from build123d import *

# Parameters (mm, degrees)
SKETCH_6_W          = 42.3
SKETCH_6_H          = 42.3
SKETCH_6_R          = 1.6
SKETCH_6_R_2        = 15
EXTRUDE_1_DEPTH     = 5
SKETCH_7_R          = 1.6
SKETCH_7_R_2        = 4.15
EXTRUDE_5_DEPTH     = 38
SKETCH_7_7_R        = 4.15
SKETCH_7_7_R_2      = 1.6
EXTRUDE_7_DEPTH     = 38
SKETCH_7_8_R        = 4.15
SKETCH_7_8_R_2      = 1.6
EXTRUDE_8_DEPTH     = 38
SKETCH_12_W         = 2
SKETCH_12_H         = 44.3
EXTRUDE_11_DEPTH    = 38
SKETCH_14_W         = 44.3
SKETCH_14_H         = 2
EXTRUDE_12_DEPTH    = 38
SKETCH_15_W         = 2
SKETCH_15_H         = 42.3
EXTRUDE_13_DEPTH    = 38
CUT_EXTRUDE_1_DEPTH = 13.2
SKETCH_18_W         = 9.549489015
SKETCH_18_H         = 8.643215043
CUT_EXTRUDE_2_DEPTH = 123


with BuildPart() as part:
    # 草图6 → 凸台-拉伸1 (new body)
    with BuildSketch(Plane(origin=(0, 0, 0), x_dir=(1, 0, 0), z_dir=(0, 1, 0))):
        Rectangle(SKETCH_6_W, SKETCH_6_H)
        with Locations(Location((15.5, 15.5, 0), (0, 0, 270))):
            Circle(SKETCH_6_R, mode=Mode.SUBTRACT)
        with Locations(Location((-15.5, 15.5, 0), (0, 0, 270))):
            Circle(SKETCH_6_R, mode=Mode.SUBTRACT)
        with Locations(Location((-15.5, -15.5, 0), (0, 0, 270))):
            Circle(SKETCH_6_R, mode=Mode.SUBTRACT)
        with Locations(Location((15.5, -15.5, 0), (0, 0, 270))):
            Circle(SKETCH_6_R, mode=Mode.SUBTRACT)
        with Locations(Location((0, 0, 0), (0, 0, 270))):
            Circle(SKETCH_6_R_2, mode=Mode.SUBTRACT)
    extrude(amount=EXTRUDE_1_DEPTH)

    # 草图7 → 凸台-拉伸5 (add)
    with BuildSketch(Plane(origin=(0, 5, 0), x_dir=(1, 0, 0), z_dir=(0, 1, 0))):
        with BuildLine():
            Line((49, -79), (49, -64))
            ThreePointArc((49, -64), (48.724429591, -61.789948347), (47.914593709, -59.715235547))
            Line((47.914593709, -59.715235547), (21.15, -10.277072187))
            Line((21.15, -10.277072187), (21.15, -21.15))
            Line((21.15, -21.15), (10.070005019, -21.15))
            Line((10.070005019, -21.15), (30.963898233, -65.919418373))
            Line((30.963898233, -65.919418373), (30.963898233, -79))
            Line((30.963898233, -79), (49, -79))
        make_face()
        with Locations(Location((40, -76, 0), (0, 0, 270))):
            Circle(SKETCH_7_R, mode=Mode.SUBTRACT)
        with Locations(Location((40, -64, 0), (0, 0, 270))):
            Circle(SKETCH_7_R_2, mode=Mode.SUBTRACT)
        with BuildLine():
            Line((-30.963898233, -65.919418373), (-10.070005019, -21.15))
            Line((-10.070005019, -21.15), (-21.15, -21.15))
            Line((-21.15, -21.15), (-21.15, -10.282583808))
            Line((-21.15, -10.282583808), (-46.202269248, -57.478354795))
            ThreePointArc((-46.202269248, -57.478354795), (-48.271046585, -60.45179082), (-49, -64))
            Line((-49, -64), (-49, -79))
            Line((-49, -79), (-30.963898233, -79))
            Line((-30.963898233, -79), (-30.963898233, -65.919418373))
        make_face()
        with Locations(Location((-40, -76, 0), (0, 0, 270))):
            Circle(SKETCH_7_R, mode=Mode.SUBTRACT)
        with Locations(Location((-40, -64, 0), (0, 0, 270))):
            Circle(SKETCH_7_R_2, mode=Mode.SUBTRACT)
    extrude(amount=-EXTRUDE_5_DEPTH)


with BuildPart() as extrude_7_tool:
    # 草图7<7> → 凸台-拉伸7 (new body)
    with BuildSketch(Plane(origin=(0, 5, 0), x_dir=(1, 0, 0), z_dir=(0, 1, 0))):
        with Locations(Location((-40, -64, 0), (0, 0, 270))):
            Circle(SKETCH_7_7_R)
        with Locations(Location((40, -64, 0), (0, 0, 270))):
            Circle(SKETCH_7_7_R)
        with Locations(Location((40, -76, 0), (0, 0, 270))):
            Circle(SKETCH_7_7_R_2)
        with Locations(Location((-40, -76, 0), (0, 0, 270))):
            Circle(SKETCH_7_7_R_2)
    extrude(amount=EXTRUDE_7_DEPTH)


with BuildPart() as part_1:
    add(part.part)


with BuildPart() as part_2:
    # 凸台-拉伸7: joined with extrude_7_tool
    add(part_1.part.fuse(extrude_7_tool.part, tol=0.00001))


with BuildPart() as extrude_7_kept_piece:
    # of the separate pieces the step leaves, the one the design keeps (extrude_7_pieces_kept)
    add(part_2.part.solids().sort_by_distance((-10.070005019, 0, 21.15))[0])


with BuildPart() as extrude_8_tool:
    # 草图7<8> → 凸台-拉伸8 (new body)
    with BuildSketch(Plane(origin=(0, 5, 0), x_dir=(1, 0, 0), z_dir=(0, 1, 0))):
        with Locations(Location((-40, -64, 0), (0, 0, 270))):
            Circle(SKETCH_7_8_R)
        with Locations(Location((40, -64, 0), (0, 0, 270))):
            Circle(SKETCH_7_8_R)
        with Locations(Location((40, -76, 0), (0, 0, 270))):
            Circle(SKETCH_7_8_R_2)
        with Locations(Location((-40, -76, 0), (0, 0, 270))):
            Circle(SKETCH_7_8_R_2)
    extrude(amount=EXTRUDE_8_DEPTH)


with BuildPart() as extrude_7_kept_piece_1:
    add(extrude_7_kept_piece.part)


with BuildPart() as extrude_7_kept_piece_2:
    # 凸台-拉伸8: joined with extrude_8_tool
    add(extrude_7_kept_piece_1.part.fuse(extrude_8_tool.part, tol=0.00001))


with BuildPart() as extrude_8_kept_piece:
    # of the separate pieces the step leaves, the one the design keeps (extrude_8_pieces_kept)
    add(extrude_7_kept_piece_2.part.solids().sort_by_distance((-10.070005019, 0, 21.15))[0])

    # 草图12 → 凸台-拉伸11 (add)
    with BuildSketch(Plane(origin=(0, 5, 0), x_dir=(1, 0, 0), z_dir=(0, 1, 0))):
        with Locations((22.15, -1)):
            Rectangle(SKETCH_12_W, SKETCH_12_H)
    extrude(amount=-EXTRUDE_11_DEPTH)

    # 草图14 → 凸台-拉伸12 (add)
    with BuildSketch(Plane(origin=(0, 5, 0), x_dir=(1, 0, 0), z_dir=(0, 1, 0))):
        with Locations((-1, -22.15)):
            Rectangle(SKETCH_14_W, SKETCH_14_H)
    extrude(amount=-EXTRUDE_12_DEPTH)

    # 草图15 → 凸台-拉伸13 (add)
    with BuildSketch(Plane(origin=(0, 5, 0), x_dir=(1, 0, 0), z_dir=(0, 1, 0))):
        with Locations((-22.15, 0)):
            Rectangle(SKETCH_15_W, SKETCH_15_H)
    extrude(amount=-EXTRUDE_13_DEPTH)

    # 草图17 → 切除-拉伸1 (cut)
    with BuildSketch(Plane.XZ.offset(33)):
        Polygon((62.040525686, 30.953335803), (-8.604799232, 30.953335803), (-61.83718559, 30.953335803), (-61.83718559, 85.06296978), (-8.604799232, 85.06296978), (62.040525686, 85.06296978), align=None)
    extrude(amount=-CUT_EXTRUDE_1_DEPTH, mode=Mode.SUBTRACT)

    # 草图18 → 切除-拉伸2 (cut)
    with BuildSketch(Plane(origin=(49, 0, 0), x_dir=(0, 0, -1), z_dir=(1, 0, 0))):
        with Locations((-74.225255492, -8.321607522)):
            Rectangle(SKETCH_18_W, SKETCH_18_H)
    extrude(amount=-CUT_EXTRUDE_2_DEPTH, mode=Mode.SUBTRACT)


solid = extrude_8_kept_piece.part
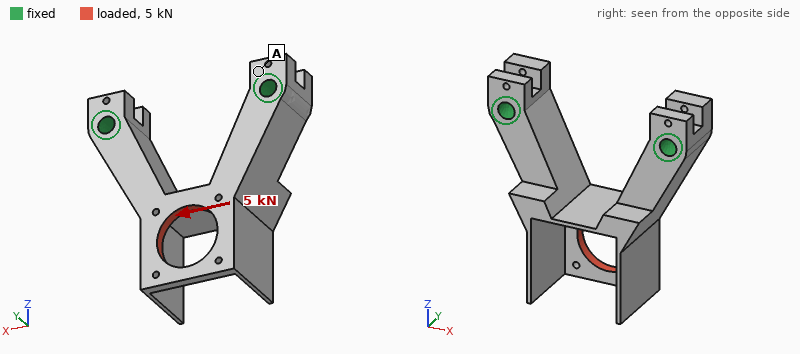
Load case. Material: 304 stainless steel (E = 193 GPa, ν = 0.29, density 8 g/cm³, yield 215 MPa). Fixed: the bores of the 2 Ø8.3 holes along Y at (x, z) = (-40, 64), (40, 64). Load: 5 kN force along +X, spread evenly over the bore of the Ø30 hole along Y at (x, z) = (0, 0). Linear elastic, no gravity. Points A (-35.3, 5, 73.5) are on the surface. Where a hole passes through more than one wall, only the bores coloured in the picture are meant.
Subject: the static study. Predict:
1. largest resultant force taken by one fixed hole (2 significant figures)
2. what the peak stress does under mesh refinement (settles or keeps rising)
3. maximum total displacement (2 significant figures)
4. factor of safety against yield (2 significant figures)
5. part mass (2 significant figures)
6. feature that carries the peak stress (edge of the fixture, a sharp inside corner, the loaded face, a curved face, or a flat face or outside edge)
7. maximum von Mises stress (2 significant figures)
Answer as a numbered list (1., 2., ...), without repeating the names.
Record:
1. 3.9 kN
2. settles
3. 76 µm
4. 1.0
5. 520 g
6. the loaded face
7. 210 MPa
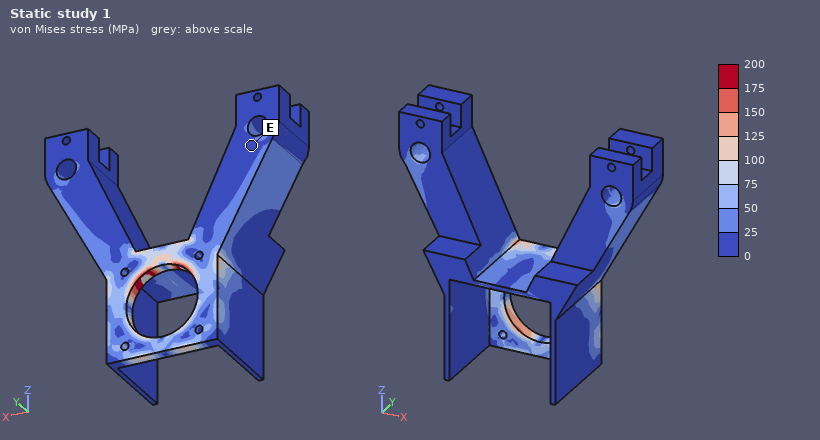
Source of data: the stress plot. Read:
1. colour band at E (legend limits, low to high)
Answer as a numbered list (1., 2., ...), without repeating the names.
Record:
1. 0 to 25 MPa
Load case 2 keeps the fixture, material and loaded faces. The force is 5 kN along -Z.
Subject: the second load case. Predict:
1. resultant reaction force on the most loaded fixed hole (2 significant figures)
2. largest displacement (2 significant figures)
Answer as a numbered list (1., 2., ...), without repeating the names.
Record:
1. 2.7 kN
2. 31 µm
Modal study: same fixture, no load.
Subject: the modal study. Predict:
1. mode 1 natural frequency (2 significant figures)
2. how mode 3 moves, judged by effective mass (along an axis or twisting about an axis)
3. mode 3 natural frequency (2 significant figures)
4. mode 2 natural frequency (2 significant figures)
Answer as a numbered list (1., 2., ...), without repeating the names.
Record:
1. 2400 Hz
2. along Y
3. 3400 Hz
4. 2400 Hz
